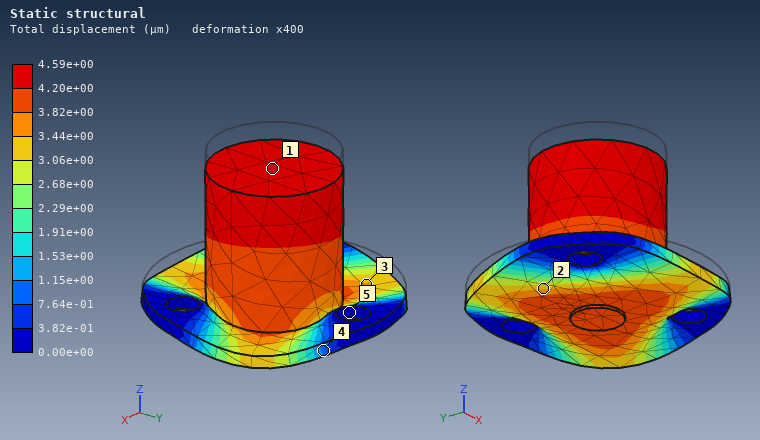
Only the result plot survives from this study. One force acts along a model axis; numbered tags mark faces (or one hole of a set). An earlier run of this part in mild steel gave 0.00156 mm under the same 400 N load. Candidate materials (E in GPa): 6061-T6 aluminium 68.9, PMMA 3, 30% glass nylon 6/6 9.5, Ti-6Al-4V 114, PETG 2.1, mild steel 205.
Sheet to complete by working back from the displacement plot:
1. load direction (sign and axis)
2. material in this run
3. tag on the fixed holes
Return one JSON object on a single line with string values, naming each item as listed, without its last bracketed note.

{"load direction": "-Z", "material in this run": "6061-T6 aluminium", "tag on the fixed holes": "5"}
